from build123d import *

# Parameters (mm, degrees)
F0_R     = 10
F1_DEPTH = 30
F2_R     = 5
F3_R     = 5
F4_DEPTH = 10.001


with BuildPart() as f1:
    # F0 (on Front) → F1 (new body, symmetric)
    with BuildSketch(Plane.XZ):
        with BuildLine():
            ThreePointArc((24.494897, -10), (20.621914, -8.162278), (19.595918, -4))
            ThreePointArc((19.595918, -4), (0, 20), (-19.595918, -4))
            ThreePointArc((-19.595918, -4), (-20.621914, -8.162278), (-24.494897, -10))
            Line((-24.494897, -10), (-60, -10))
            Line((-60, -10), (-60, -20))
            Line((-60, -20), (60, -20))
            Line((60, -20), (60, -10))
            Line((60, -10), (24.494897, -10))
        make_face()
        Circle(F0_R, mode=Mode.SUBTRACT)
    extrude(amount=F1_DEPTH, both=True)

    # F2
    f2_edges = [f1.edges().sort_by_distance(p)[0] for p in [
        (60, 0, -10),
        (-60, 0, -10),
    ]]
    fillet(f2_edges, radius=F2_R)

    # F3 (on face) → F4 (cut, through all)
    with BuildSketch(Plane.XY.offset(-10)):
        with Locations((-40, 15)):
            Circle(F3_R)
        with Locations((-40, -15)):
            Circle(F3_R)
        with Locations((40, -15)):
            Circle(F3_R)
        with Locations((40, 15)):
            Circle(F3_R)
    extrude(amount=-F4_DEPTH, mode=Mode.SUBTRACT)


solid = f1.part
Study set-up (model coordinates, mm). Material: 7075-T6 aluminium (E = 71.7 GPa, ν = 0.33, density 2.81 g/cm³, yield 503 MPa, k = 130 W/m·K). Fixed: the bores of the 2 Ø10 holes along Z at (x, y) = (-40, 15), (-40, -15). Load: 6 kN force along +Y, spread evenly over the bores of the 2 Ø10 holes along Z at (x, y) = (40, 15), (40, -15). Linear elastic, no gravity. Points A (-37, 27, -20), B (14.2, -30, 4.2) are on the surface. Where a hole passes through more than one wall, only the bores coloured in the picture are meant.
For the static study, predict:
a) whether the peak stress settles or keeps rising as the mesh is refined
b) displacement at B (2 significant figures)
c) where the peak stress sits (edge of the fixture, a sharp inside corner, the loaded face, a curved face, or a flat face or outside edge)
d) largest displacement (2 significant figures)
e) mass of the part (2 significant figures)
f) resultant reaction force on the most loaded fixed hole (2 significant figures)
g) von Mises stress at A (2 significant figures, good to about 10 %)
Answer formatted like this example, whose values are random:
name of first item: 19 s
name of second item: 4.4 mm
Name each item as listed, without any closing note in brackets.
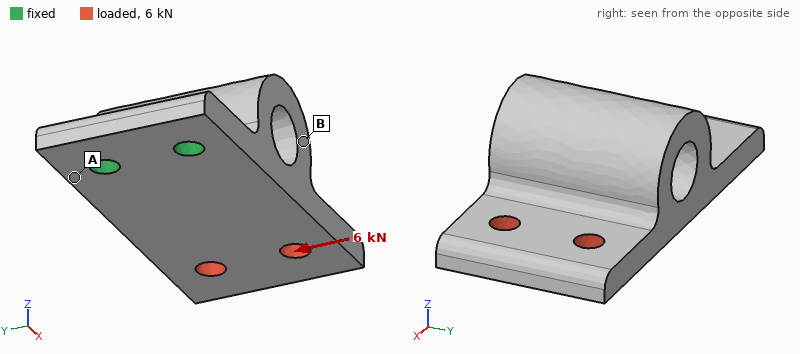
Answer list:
whether the peak stress settles or keeps rising as the mesh is refined: keeps rising
displacement at B: 0.074 mm
where the peak stress sits: edge of the fixture
largest displacement: 0.16 mm
mass of the part: 310 g
resultant reaction force on the most loaded fixed hole: 13 kN
von Mises stress at A: 34 MPa
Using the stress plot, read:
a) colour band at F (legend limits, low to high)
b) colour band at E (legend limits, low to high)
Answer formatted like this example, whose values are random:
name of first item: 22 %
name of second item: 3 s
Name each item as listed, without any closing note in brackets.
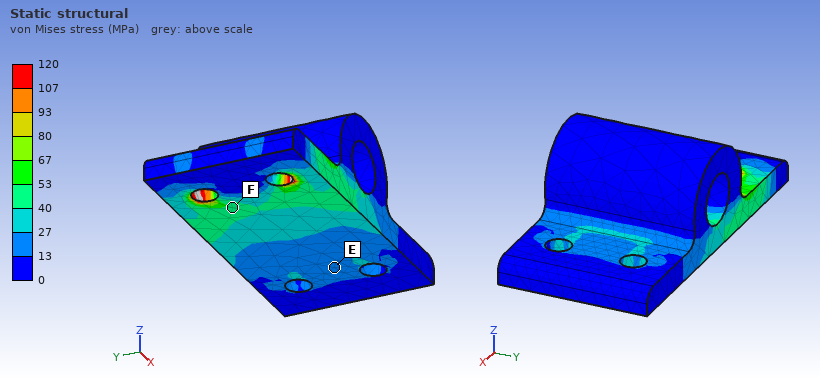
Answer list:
colour band at F: 40 to 53 MPa
colour band at E: 13 to 27 MPa
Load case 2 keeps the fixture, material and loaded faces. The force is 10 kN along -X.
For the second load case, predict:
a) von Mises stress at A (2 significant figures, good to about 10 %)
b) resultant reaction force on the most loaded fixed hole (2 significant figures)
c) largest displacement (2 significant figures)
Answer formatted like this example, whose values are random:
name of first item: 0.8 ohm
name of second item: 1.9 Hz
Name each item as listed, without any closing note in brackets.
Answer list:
von Mises stress at A: 8.5 MPa
resultant reaction force on the most loaded fixed hole: 5.0 kN
largest displacement: 39 µm
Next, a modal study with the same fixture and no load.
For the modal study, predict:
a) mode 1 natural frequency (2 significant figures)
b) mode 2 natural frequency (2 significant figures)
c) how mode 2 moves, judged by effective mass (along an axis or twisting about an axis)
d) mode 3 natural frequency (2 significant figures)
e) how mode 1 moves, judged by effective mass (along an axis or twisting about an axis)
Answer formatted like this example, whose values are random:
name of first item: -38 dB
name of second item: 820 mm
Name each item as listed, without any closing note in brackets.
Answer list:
mode 1 natural frequency: 890 Hz
mode 2 natural frequency: 3400 Hz
how mode 2 moves, judged by effective mass: along Y
mode 3 natural frequency: 3700 Hz
how mode 1 moves, judged by effective mass: along Z
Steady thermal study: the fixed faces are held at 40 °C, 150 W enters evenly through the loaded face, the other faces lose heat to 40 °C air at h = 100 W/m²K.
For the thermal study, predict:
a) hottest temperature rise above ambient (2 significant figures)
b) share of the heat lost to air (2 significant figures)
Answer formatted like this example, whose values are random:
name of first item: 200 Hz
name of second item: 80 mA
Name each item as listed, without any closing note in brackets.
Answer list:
hottest temperature rise above ambient: 85 K
share of the heat lost to air: 54 %
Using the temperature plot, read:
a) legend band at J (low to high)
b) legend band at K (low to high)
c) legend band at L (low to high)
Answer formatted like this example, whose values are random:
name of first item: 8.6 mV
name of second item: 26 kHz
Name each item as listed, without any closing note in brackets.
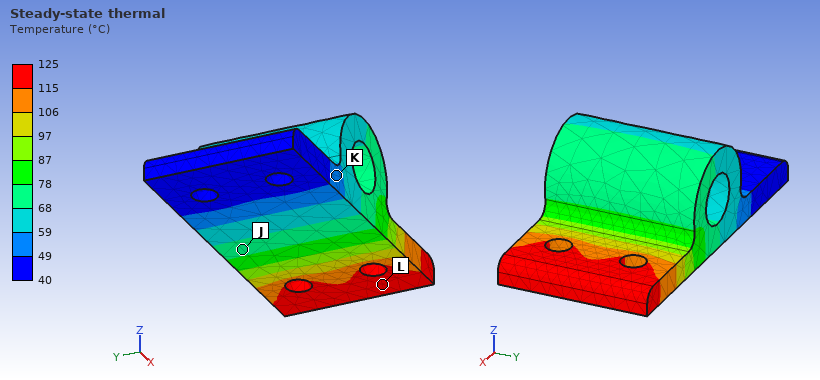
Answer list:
legend band at J: 68 to 78 °C
legend band at K: 49 to 59 °C
legend band at L: 115 to 125 °C
